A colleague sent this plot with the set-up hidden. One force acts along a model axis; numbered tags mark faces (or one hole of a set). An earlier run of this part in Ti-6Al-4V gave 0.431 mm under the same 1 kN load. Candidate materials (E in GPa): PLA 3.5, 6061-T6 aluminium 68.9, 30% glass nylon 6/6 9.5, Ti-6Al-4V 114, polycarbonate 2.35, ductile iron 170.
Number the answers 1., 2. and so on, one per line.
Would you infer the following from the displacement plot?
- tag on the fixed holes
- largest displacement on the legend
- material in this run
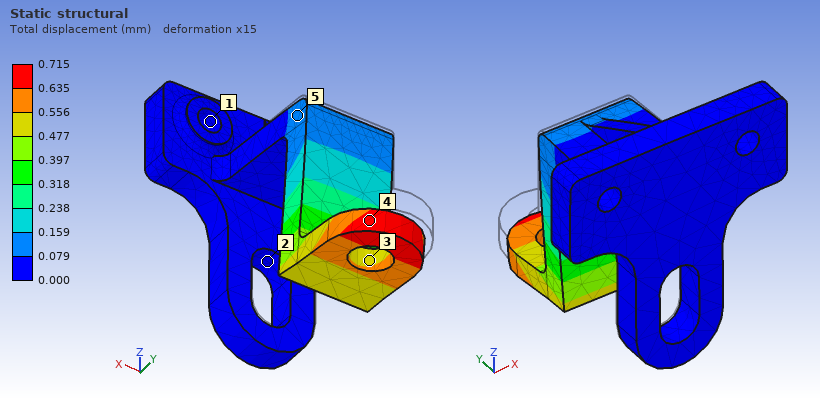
1. 1
2. 0.715 mm
3. 6061-T6 aluminium
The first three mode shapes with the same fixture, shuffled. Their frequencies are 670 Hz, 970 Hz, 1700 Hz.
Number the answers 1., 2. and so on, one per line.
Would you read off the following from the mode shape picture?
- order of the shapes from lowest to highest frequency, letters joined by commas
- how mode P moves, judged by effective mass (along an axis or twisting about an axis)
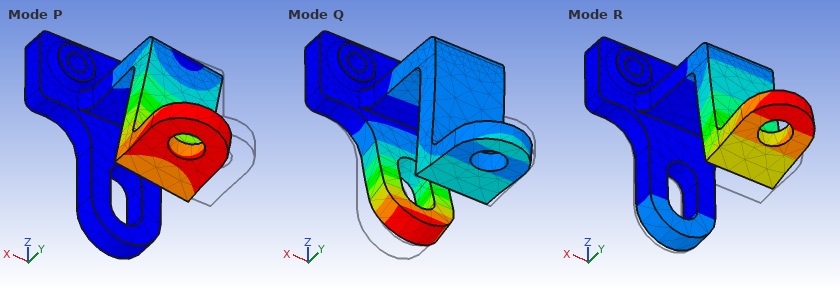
1. R, P, Q
2. along X
